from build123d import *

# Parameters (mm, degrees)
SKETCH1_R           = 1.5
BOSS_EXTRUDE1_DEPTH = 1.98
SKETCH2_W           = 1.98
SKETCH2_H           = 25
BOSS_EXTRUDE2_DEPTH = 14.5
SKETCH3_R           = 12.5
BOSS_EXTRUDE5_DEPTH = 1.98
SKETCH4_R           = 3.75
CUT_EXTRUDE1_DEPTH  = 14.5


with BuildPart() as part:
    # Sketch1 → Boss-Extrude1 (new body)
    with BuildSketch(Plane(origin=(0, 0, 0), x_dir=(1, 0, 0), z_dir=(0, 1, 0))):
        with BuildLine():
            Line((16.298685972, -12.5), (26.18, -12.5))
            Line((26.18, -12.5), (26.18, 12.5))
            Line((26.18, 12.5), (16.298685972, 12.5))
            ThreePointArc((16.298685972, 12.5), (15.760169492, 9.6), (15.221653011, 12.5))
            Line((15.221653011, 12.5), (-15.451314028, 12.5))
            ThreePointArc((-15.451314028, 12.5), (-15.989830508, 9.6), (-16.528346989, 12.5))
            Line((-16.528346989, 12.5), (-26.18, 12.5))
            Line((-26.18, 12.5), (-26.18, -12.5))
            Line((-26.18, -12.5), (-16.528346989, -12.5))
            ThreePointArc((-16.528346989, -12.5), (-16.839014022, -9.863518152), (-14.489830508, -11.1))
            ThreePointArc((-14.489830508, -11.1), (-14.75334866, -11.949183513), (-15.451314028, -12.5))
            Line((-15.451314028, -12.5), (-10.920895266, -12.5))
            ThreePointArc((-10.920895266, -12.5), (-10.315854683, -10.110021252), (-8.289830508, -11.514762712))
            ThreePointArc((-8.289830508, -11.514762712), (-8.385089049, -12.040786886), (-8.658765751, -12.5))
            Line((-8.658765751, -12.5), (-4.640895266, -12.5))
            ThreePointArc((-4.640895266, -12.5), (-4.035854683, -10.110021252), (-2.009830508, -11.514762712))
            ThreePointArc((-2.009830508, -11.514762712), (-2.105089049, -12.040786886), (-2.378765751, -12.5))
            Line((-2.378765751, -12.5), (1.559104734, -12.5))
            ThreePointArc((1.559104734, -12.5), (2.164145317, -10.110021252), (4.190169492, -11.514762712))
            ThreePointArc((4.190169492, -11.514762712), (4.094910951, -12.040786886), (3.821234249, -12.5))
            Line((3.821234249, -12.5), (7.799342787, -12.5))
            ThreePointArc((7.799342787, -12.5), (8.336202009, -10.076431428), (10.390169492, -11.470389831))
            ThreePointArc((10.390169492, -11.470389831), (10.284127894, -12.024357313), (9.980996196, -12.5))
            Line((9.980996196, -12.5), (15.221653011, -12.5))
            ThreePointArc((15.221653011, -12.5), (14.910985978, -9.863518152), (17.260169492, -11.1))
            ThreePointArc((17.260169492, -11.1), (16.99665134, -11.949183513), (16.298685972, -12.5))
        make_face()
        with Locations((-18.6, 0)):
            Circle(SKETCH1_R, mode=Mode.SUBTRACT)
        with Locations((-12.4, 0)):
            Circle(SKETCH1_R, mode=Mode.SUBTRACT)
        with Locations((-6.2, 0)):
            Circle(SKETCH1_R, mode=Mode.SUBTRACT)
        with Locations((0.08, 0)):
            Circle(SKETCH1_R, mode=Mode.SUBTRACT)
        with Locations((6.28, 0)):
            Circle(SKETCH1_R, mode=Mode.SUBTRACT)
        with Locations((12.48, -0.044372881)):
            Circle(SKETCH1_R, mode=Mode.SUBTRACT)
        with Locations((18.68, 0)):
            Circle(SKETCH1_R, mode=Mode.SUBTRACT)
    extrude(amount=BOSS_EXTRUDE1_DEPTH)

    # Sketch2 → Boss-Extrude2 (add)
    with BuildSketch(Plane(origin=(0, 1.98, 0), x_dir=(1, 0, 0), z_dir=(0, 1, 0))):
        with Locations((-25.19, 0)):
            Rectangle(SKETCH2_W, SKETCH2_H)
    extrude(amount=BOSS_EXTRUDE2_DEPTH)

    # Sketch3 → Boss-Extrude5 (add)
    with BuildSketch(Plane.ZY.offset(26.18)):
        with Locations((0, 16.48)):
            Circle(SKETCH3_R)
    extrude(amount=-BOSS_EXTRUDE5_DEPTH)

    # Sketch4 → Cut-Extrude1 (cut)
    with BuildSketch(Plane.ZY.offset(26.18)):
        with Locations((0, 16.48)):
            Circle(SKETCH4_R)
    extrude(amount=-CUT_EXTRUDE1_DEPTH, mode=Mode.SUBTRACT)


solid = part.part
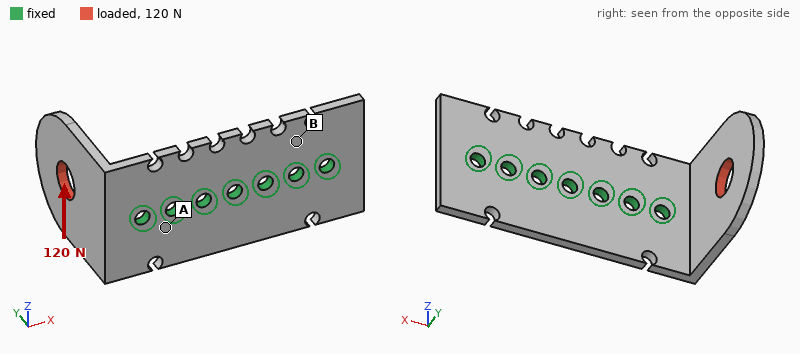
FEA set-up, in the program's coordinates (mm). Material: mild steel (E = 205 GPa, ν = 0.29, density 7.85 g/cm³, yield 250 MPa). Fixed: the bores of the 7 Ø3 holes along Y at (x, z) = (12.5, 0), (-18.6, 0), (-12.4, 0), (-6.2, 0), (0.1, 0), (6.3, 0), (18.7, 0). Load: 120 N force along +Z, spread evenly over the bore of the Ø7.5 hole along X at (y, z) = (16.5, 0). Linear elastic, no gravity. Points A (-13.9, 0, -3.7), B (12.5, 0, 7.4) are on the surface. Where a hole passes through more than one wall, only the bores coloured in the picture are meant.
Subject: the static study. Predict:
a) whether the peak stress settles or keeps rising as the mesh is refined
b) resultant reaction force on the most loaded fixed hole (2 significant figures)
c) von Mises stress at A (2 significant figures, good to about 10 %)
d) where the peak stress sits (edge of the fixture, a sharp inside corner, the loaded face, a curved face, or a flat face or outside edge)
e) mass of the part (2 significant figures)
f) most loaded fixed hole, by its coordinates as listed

keeps rising
140 N
41 MPa
edge of the fixture
28 g
(-18.6, 0)
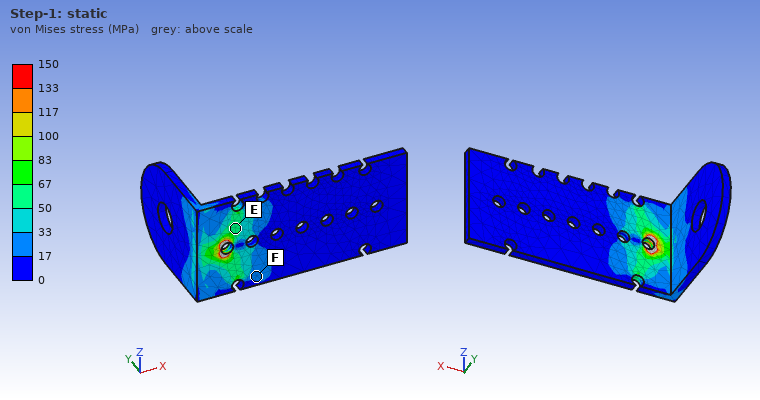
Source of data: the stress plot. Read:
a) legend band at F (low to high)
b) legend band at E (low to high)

17 to 33 MPa
50 to 67 MPa
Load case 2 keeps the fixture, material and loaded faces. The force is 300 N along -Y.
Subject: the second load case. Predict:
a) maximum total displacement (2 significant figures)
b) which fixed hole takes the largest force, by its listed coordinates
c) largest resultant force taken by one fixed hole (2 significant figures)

65 µm
(-18.6, 0)
380 N
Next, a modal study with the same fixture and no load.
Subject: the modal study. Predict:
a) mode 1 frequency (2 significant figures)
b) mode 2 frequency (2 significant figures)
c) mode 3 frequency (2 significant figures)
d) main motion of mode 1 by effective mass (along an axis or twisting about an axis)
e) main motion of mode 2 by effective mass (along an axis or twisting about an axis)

1800 Hz
2800 Hz
6300 Hz
along X
along Z
